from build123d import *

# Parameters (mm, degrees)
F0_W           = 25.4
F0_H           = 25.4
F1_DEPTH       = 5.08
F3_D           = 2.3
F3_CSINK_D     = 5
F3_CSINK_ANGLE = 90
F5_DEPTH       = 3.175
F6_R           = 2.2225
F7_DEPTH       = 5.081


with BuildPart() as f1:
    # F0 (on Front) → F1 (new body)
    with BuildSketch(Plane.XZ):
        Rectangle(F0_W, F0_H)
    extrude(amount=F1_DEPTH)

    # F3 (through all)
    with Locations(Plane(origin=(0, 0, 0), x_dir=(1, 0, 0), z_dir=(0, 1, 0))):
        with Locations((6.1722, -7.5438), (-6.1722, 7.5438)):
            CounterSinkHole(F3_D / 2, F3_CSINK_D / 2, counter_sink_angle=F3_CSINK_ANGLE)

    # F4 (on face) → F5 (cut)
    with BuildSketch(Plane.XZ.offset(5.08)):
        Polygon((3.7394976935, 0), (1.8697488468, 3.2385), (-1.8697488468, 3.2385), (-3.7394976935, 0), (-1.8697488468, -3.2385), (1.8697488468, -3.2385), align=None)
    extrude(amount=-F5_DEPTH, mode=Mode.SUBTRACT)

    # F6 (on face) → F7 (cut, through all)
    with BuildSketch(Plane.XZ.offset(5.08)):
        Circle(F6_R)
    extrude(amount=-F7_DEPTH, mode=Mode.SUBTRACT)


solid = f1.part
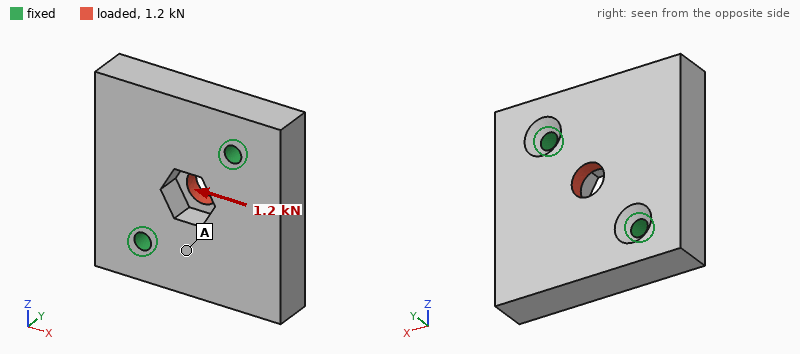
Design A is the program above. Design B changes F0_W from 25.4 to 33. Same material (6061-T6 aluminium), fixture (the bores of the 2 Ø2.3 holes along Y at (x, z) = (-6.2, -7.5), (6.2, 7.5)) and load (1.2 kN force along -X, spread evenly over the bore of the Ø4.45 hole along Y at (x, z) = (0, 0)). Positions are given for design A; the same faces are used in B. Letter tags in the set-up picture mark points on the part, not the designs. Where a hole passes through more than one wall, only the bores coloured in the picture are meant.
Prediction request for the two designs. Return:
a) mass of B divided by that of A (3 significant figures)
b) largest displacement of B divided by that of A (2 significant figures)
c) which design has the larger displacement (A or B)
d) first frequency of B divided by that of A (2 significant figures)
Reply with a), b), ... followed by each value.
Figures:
a) 1.32
b) 1.1
c) B
d) 0.76
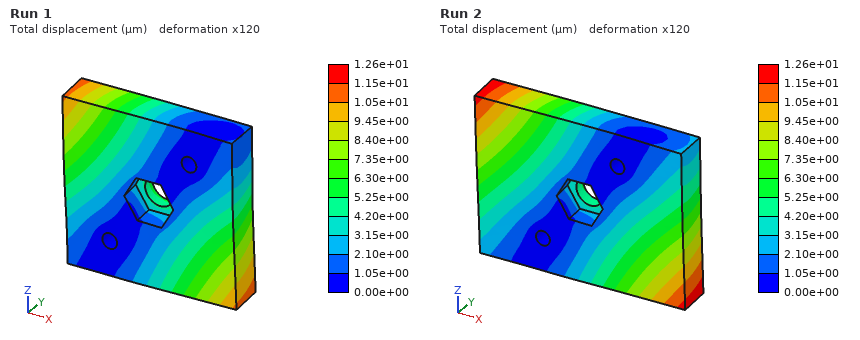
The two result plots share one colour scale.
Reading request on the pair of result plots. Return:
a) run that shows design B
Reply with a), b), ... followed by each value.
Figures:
a) Run 2
